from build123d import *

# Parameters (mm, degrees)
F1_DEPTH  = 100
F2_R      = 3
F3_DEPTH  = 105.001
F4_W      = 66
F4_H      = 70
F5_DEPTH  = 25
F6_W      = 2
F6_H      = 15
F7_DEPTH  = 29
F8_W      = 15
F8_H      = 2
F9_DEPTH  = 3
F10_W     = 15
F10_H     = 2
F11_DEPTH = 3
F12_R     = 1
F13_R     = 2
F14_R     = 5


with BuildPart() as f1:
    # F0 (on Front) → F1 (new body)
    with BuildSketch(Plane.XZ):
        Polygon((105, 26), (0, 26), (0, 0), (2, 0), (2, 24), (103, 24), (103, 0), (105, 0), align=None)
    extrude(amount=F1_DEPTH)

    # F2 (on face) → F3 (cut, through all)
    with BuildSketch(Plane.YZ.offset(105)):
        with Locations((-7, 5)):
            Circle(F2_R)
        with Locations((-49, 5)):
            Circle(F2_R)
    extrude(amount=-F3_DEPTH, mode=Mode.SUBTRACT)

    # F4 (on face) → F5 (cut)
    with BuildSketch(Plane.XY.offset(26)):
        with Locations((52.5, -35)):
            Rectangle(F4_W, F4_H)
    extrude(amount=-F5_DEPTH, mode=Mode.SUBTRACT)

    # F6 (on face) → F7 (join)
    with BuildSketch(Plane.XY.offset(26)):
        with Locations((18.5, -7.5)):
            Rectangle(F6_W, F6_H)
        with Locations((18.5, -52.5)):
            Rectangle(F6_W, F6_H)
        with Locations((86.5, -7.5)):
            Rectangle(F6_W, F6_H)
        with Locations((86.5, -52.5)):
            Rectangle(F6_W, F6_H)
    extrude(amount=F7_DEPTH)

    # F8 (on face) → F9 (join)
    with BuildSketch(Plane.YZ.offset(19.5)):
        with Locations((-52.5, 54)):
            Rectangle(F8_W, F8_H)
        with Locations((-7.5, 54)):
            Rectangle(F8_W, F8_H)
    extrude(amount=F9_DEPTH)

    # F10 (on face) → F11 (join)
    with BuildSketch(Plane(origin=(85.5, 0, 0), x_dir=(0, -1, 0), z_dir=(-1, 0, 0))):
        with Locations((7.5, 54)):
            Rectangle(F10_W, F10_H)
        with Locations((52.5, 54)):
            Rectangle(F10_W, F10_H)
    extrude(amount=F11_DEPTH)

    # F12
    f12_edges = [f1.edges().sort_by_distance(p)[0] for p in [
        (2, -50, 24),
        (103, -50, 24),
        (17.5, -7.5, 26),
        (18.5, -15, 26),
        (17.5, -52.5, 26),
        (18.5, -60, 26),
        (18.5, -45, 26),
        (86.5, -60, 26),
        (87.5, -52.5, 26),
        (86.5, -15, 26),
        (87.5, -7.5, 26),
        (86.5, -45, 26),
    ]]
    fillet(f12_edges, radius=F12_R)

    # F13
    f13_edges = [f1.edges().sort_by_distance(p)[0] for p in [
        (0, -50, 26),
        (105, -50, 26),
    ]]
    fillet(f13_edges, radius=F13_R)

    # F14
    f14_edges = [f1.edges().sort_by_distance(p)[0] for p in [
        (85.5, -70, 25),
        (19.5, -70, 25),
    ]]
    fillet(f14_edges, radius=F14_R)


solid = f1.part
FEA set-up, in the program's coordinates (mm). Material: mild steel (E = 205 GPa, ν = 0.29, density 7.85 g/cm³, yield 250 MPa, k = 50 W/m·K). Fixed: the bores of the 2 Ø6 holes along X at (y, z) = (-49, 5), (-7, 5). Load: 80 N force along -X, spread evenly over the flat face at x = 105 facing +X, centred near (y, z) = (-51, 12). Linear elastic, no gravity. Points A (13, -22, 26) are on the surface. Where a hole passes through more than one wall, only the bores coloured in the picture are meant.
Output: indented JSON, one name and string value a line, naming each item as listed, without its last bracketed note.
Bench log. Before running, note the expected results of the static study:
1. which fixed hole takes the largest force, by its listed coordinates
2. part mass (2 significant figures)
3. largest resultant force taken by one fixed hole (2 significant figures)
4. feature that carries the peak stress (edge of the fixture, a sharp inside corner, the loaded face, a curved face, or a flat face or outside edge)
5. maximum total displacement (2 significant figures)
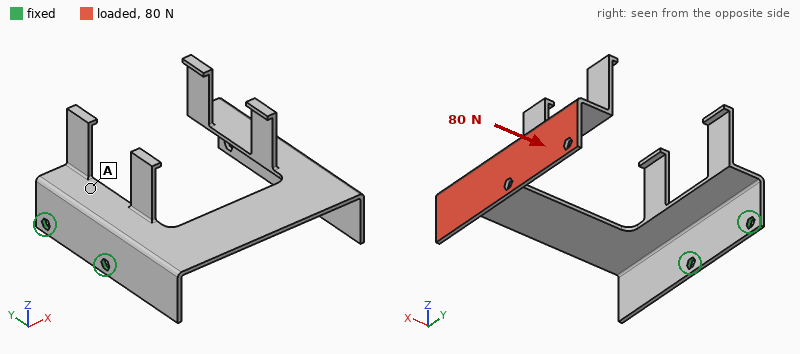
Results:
{
  "which fixed hole takes the largest force, by its listed coordinates": "(-49, 5)",
  "part mass": "200 g",
  "largest resultant force taken by one fixed hole": "72 N",
  "feature that carries the peak stress": "a curved face",
  "maximum total displacement": "1.5 mm"
}
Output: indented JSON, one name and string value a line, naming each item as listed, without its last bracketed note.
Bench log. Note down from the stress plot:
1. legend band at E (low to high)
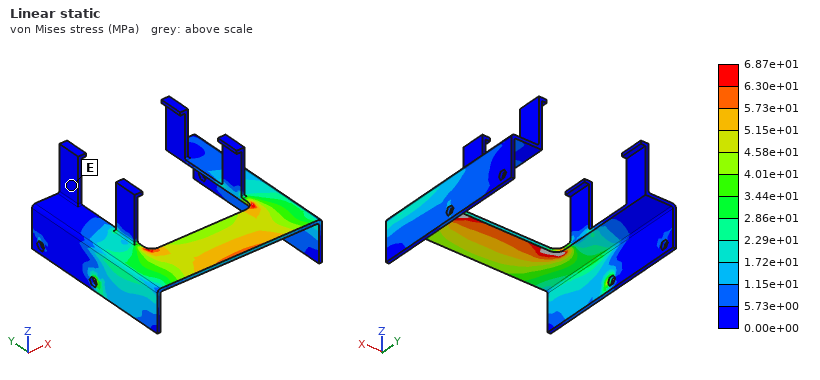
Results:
{
  "legend band at E": "0.00e+00 to 5.73e+00 MPa"
}
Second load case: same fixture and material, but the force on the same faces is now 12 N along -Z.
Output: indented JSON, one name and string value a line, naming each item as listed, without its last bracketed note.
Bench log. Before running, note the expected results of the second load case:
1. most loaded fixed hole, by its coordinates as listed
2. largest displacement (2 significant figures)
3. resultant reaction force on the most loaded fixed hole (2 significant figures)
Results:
{
  "most loaded fixed hole, by its coordinates as listed": "(-49, 5)",
  "largest displacement": "1.8 mm",
  "resultant reaction force on the most loaded fixed hole": "14 N"
}
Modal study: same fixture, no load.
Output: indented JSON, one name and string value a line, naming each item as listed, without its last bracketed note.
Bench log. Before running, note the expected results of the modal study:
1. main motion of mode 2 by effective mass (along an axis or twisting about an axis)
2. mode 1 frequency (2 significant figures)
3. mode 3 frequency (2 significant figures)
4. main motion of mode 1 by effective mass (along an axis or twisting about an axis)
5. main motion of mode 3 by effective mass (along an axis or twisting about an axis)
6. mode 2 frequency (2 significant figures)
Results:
{
  "main motion of mode 2 by effective mass": "twisting about X",
  "mode 1 frequency": "51 Hz",
  "mode 3 frequency": "240 Hz",
  "main motion of mode 1 by effective mass": "along Z",
  "main motion of mode 3 by effective mass": "along Y",
  "mode 2 frequency": "140 Hz"
}
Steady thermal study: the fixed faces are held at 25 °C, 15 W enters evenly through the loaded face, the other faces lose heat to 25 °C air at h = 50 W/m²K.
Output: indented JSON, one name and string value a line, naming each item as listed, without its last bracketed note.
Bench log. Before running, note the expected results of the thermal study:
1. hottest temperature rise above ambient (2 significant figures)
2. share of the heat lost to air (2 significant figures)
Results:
{
  "hottest temperature rise above ambient": "46 K",
  "share of the heat lost to air": "100 %"
}
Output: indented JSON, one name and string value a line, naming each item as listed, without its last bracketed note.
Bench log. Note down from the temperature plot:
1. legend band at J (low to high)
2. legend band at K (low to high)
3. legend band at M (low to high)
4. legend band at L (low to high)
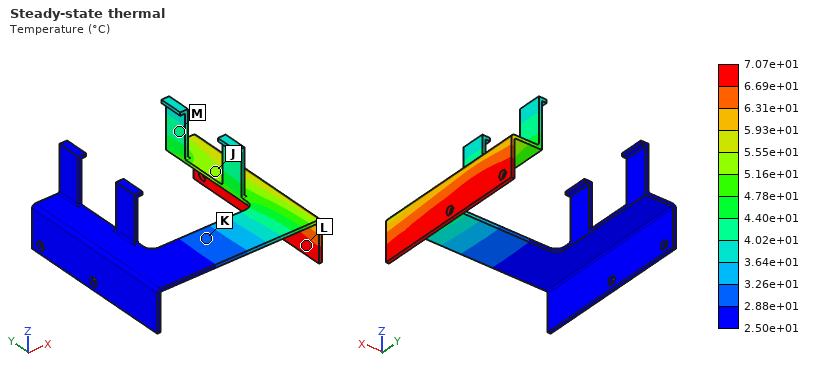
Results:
{
  "legend band at J": "5.16e+01 to 5.55e+01 °C",
  "legend band at K": "2.88e+01 to 3.26e+01 °C",
  "legend band at M": "4.02e+01 to 4.40e+01 °C",
  "legend band at L": "6.69e+01 to 7.07e+01 °C"
}
